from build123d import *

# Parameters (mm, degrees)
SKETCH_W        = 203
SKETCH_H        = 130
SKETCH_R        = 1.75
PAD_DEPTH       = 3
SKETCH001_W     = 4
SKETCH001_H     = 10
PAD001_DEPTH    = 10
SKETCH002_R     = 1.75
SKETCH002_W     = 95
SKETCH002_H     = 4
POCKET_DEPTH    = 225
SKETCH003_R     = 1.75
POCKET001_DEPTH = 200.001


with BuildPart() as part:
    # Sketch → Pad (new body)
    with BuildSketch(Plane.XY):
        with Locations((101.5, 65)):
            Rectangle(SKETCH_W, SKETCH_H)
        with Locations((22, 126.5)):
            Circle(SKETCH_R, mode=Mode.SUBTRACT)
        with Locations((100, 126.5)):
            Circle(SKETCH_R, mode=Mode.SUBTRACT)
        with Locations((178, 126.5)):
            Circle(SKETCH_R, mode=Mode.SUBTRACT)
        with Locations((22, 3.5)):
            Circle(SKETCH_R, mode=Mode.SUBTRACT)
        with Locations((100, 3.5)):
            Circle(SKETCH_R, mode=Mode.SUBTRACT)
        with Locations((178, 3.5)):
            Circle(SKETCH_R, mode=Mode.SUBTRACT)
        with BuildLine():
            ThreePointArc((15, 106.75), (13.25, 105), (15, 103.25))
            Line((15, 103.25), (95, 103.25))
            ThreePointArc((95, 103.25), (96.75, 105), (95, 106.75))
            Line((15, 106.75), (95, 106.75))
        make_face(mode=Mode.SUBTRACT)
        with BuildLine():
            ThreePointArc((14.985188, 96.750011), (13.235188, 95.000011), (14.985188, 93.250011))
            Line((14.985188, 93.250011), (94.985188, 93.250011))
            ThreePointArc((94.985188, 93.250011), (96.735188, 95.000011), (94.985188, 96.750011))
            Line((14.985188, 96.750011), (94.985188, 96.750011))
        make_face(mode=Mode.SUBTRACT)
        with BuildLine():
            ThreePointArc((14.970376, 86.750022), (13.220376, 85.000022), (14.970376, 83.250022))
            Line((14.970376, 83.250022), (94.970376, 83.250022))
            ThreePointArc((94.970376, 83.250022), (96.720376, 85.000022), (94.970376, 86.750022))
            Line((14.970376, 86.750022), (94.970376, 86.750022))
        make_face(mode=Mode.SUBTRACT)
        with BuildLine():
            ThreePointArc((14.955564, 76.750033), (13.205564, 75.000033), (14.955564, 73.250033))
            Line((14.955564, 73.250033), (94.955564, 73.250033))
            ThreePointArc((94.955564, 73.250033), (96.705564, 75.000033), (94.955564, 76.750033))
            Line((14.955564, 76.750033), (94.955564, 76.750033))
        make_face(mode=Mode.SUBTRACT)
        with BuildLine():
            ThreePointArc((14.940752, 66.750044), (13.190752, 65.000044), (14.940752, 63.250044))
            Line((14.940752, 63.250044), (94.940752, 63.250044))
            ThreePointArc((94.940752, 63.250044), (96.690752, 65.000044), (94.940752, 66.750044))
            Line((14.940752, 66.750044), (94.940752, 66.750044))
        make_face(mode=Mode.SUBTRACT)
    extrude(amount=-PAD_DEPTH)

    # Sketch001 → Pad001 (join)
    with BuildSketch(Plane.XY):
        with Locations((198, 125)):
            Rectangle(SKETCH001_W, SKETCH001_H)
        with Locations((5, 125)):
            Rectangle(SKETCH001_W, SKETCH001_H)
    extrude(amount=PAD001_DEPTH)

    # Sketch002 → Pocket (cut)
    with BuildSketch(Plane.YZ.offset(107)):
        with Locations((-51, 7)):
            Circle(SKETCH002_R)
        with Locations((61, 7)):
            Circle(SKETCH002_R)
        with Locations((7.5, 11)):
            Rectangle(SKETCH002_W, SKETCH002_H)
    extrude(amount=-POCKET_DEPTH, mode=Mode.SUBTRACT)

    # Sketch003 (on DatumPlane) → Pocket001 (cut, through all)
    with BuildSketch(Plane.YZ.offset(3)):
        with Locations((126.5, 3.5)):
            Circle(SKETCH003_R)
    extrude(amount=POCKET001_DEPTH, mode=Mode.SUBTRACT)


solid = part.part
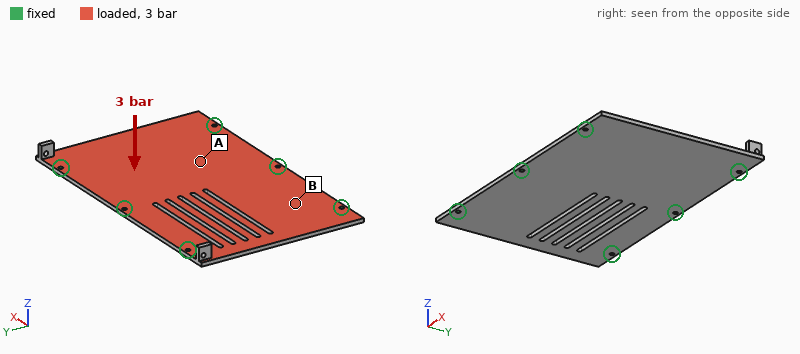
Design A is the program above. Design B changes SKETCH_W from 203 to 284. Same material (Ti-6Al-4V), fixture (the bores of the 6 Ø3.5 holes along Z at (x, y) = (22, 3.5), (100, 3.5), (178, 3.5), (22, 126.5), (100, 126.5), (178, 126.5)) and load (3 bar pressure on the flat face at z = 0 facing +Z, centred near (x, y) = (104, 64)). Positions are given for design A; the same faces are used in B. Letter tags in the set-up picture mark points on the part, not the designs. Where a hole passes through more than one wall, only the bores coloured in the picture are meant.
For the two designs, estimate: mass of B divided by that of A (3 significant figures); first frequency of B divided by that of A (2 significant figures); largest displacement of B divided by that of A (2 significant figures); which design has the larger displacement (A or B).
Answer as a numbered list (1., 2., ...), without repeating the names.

1. 1.42
2. 0.60
3. 2.6
4. B
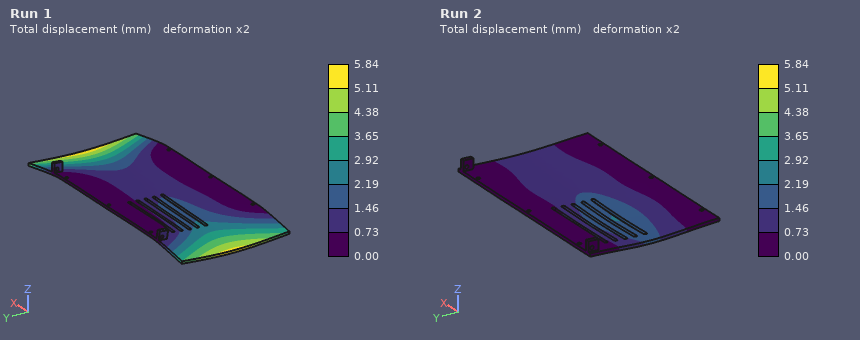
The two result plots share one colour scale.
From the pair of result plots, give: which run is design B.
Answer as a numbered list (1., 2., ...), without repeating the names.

1. Run 1
